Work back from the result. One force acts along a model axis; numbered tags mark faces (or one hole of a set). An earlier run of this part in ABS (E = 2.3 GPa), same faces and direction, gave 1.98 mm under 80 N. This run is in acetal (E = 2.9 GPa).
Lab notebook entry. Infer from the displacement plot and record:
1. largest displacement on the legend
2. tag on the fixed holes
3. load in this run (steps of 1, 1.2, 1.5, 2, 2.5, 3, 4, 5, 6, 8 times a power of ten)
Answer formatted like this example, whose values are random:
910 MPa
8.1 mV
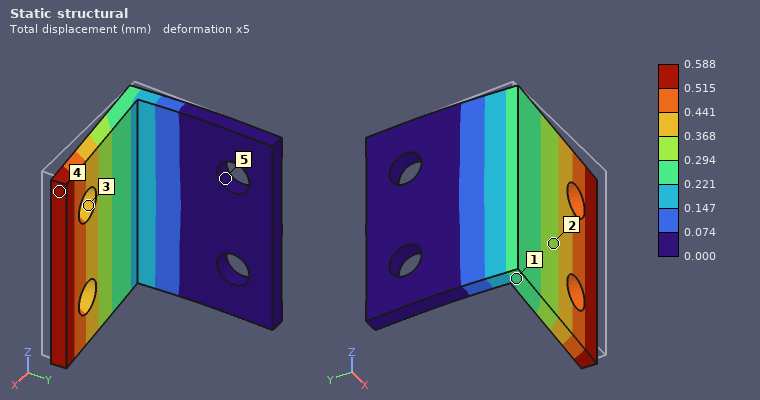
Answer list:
0.588 mm
5
30 N
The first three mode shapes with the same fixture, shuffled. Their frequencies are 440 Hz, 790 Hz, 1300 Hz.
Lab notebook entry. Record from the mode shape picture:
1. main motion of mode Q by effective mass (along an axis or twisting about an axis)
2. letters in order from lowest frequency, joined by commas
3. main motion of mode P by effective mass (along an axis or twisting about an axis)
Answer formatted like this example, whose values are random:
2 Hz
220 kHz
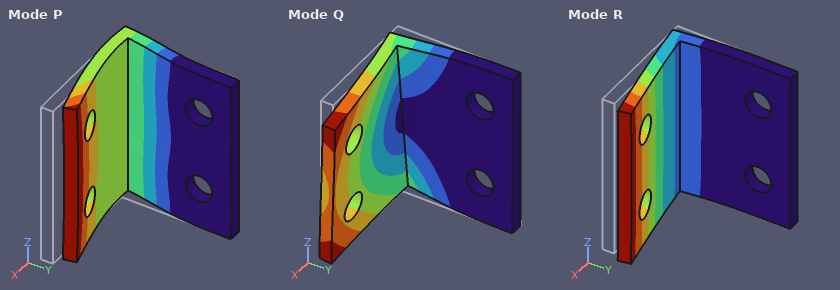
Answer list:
along Z
R, Q, P
along X
